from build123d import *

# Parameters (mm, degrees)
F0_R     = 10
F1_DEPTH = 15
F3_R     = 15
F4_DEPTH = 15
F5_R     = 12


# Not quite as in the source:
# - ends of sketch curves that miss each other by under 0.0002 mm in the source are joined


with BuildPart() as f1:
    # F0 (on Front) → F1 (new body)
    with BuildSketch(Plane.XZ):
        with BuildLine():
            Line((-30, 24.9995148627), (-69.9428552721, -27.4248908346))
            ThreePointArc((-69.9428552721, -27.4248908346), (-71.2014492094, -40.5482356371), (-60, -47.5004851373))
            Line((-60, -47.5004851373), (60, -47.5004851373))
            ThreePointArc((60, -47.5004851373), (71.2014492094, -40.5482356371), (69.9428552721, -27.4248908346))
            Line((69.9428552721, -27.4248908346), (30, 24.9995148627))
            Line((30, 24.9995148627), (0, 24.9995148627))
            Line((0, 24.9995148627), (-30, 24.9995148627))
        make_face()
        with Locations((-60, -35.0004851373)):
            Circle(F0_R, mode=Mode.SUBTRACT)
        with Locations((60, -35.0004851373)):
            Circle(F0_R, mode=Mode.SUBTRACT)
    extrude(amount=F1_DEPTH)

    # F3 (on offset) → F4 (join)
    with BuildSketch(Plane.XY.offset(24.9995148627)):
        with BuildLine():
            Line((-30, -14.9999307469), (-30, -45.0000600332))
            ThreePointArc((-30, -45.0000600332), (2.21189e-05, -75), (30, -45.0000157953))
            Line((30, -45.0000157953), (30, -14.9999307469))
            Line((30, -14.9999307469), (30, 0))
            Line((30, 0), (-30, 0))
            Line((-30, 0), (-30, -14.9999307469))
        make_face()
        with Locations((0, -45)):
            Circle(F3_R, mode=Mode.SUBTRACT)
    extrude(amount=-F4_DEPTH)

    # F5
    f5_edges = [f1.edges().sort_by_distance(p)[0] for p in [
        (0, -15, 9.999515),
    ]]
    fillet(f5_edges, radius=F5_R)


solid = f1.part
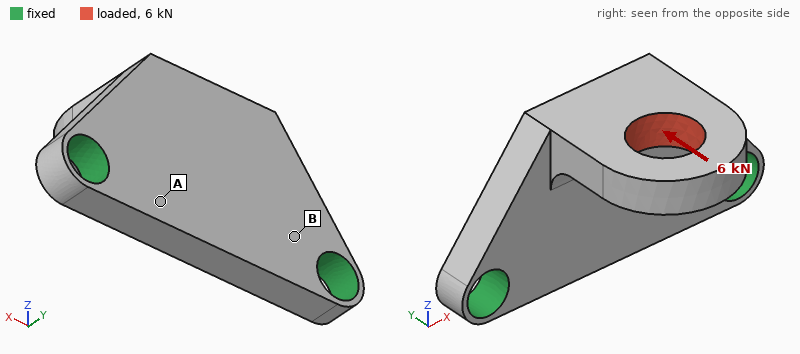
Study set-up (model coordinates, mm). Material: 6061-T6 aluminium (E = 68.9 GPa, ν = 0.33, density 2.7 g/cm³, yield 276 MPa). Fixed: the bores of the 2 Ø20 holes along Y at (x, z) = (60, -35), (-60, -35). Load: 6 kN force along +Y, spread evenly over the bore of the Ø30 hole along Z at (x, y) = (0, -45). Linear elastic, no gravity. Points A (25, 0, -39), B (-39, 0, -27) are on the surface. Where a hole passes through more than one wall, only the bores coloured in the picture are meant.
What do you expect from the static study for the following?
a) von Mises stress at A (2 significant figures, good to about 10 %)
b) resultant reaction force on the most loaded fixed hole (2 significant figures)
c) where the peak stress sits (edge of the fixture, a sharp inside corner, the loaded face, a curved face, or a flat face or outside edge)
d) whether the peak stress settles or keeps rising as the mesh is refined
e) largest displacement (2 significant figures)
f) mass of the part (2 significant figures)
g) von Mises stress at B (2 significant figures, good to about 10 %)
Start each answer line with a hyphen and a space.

- 28 MPa
- 3.0 kN
- edge of the fixture
- keeps rising
- 0.44 mm
- 410 g
- 58 MPa
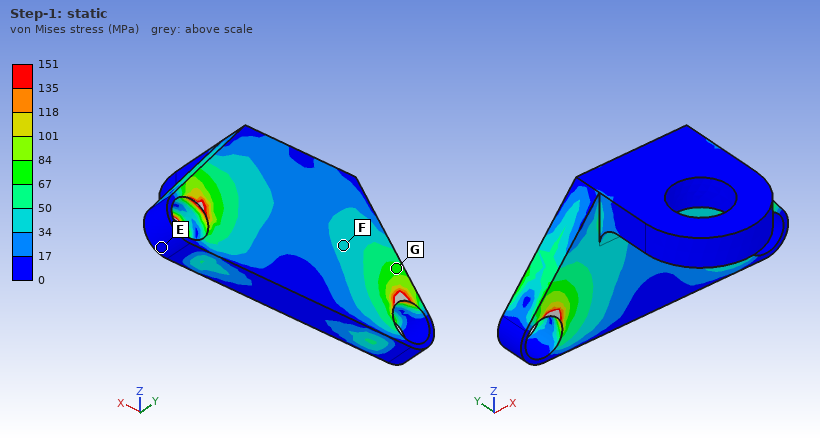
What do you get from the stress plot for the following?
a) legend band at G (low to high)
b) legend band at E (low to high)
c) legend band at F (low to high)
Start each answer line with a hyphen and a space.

- 67 to 84 MPa
- 0 to 17 MPa
- 34 to 50 MPa
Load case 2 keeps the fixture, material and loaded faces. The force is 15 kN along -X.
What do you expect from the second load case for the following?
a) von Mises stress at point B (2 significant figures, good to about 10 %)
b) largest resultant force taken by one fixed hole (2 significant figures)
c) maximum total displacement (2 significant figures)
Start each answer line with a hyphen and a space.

- 43 MPa
- 12 kN
- 0.40 mm
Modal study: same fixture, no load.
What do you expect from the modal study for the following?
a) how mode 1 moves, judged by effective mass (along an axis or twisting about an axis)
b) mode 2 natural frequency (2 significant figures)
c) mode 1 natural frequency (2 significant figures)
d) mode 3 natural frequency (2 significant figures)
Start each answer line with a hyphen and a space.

- along Y
- 3500 Hz
- 1600 Hz
- 3500 Hz
